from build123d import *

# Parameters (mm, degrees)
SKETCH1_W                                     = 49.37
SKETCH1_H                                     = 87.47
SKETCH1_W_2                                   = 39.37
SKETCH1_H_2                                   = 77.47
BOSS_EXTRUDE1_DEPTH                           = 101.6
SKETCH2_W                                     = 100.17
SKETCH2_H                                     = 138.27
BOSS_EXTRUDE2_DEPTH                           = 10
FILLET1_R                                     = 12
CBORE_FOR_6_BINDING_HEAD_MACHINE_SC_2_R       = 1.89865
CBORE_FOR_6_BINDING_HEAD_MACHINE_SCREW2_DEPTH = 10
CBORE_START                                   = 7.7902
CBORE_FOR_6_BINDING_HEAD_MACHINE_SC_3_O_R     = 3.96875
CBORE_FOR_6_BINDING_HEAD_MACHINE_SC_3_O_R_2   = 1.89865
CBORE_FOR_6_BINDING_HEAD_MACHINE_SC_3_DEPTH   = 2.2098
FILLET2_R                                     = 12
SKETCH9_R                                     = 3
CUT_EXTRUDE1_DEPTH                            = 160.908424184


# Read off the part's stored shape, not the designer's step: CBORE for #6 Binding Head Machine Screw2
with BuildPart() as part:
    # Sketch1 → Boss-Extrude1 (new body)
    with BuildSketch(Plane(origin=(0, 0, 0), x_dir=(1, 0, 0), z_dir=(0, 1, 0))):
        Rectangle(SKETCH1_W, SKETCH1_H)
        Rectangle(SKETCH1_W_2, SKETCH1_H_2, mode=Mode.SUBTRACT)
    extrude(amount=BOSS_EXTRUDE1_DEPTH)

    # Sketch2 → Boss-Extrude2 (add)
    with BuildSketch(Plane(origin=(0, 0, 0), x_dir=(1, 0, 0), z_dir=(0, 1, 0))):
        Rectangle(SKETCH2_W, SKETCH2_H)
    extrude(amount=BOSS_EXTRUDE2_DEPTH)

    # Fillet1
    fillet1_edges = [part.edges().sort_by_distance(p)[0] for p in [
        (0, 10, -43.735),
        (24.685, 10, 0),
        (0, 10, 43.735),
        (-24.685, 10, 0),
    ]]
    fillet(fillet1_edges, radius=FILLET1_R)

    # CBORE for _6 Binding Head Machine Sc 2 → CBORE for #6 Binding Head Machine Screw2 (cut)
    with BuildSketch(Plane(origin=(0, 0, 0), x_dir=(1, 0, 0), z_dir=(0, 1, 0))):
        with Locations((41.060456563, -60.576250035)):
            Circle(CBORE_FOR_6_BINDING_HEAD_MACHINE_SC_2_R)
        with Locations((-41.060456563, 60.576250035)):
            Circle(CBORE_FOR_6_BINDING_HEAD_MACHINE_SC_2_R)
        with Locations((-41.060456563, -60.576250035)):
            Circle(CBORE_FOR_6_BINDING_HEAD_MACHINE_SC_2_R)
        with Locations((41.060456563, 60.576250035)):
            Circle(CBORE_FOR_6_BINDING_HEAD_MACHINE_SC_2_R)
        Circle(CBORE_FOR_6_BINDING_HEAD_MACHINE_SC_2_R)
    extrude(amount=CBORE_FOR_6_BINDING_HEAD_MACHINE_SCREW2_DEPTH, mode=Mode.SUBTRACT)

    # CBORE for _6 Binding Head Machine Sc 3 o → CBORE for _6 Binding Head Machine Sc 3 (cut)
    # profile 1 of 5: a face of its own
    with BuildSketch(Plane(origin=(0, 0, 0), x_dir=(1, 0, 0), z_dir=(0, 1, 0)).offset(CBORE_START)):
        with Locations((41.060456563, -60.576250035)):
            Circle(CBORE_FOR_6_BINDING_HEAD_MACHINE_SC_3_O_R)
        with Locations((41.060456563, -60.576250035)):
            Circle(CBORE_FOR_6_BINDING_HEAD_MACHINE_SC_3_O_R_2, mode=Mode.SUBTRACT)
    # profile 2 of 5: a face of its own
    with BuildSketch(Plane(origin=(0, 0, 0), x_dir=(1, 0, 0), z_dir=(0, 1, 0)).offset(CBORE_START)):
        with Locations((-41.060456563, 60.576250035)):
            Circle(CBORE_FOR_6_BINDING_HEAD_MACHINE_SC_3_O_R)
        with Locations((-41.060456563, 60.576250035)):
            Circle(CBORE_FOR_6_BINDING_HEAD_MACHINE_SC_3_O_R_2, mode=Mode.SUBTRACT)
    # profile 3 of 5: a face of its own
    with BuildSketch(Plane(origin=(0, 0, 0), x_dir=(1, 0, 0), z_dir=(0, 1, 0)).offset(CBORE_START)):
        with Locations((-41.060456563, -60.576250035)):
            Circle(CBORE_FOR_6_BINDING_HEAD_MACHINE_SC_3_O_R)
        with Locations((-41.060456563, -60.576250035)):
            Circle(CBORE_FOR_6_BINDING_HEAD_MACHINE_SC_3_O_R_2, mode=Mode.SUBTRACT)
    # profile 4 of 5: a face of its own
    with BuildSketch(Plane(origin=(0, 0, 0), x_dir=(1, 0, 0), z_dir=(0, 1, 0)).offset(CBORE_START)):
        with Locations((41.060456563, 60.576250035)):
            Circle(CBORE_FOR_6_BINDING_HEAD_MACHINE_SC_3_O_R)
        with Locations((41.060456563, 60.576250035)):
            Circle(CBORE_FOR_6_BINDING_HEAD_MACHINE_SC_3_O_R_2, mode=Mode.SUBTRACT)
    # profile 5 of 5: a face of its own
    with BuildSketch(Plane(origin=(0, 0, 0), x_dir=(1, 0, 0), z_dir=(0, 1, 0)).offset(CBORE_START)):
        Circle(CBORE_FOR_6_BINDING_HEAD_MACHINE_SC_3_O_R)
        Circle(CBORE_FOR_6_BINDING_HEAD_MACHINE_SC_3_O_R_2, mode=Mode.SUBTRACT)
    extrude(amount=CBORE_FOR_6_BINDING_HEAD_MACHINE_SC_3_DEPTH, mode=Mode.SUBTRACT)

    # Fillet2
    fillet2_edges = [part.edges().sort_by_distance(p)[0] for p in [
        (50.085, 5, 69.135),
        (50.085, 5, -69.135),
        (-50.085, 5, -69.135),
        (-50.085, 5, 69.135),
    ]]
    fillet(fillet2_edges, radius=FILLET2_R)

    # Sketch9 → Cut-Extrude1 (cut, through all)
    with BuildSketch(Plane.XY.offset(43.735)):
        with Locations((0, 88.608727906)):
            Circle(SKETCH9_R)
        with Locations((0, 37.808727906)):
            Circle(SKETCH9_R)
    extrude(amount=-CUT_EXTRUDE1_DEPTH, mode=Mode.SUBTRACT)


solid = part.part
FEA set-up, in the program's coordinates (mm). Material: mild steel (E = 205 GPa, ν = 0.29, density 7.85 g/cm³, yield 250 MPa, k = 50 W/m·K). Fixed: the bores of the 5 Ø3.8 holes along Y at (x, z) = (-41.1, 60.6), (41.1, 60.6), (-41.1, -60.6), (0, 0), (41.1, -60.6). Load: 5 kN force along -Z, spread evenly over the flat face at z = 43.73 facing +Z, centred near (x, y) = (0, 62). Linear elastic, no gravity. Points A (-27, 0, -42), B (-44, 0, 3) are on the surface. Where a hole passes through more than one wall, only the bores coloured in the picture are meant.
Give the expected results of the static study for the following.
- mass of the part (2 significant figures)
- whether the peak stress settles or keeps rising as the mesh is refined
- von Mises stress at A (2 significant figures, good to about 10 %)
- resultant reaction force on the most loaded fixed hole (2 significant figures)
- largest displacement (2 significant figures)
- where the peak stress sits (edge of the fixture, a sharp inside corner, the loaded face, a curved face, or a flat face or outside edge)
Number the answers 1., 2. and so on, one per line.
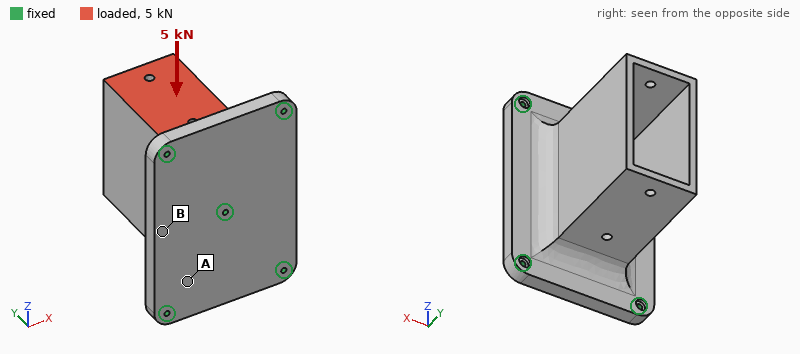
1. 2.0 kg
2. keeps rising
3. 11 MPa
4. 1.8 kN
5. 39 µm
6. edge of the fixture
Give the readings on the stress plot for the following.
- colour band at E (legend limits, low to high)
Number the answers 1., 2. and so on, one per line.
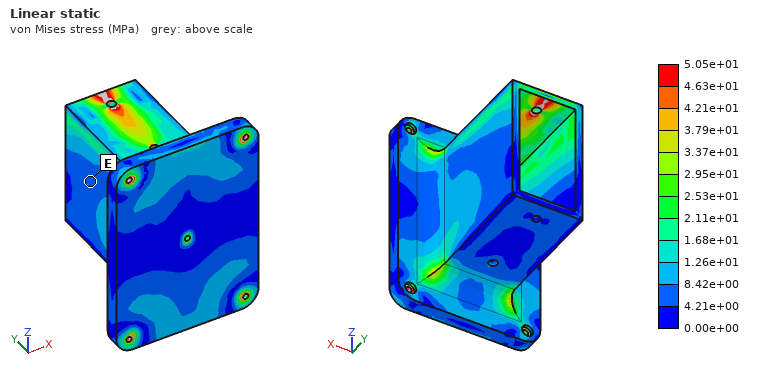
1. 4.21e+00 to 8.42e+00 MPa
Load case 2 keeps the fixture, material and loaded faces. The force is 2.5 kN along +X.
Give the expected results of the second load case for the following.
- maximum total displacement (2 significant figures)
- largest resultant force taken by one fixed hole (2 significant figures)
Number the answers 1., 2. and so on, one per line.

1. 35 µm
2. 1.8 kN
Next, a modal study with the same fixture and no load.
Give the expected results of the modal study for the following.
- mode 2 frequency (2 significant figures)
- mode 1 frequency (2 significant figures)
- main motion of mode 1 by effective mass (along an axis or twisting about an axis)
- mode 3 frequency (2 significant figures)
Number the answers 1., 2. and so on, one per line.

1. 2900 Hz
2. 2000 Hz
3. along X
4. 2900 Hz
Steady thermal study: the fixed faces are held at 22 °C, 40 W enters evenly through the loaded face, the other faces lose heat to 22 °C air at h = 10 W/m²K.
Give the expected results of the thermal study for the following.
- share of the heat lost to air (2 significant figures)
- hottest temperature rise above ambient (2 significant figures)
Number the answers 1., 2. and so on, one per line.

1. 30 %
2. 57 K
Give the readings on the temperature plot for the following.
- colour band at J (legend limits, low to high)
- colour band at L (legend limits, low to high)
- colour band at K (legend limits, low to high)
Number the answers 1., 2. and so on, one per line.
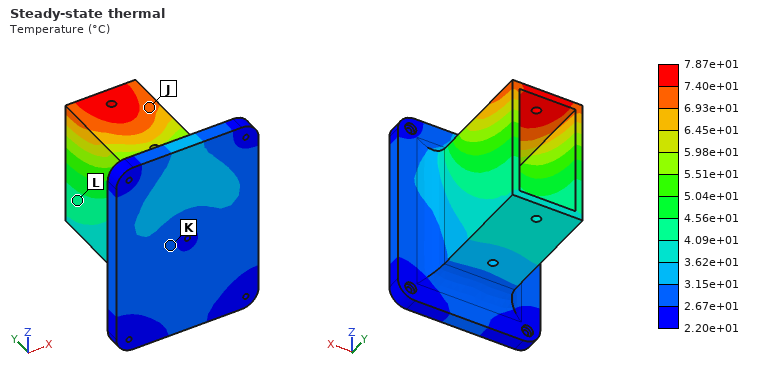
1. 6.93e+01 to 7.40e+01 °C
2. 4.09e+01 to 4.56e+01 °C
3. 2.67e+01 to 3.15e+01 °C
